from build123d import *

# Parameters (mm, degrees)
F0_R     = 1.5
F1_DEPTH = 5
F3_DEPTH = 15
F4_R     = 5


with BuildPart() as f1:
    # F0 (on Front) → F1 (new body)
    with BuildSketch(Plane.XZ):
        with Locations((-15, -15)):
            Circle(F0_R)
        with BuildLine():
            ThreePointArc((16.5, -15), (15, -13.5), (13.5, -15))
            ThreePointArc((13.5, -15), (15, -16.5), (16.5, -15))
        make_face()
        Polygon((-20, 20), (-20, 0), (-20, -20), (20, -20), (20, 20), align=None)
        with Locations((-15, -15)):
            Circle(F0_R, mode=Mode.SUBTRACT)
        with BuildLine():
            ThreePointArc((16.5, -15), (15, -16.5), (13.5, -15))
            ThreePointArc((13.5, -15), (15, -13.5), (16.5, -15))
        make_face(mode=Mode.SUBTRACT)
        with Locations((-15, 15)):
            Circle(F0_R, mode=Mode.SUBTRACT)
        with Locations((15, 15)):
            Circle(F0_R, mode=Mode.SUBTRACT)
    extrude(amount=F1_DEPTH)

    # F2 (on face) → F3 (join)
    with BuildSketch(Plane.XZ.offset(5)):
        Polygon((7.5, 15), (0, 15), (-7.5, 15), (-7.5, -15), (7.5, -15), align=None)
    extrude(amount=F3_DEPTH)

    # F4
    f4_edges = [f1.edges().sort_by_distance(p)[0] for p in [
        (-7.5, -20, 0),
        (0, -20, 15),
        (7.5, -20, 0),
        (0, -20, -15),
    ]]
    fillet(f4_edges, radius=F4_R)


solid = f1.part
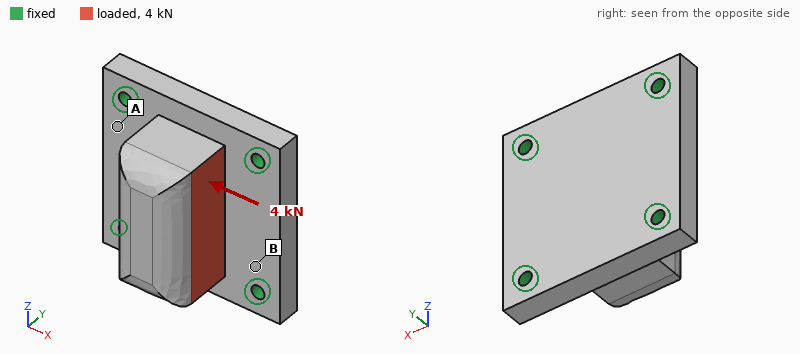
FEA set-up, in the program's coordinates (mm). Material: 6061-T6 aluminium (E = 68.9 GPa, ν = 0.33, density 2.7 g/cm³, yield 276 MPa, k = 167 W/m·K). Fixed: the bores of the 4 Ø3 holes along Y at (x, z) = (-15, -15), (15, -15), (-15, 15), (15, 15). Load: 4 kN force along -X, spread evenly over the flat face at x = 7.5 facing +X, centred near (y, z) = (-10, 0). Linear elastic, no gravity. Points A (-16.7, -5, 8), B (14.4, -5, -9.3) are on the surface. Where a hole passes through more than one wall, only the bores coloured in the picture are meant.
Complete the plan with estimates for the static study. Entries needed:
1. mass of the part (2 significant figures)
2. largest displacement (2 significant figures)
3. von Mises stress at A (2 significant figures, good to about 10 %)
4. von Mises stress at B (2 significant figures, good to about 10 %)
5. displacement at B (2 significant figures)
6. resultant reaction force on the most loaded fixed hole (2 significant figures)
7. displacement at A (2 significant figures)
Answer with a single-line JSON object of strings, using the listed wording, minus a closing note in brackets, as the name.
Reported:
{"mass of the part": "38 g", "largest displacement": "21 µm", "von Mises stress at A": "6.8 MPa", "von Mises stress at B": "13 MPa", "displacement at B": "3.9 µm", "resultant reaction force on the most loaded fixed hole": "1.2 kN", "displacement at A": "3.9 µm"}
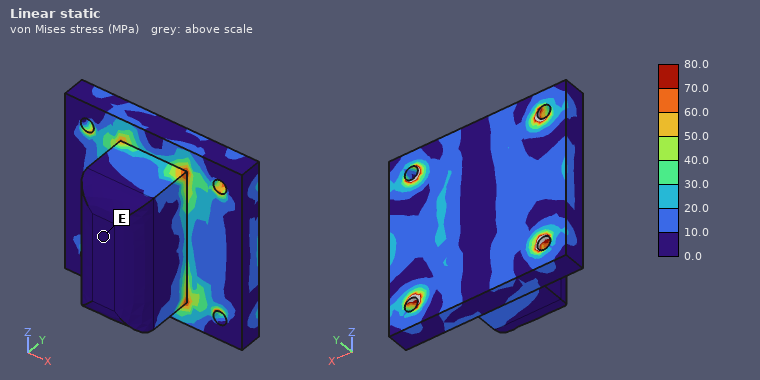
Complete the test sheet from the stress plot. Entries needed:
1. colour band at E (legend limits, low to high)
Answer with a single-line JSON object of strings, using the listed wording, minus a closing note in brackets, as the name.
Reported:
{"colour band at E": "0.0 to 10.0 MPa"}
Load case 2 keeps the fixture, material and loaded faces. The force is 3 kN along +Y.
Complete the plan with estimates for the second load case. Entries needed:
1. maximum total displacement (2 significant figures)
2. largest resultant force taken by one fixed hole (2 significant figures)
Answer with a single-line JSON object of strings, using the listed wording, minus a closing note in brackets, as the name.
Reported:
{"maximum total displacement": "24 µm", "largest resultant force taken by one fixed hole": "1.2 kN"}
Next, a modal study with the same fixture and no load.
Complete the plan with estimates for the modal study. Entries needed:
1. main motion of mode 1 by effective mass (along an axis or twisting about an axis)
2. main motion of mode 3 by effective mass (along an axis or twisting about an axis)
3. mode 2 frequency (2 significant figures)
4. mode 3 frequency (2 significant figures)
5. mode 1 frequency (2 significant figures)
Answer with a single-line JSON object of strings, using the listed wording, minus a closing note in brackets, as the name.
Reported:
{"main motion of mode 1 by effective mass": "along Y", "main motion of mode 3 by effective mass": "along X", "mode 2 frequency": "15 kHz", "mode 3 frequency": "16 kHz", "mode 1 frequency": "14 kHz"}
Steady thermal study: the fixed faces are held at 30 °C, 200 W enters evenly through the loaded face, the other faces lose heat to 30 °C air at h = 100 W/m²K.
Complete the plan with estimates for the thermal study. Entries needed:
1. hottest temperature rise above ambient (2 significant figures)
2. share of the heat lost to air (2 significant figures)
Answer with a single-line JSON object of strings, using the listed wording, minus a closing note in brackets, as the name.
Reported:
{"hottest temperature rise above ambient": "71 K", "share of the heat lost to air": "7.1 %"}
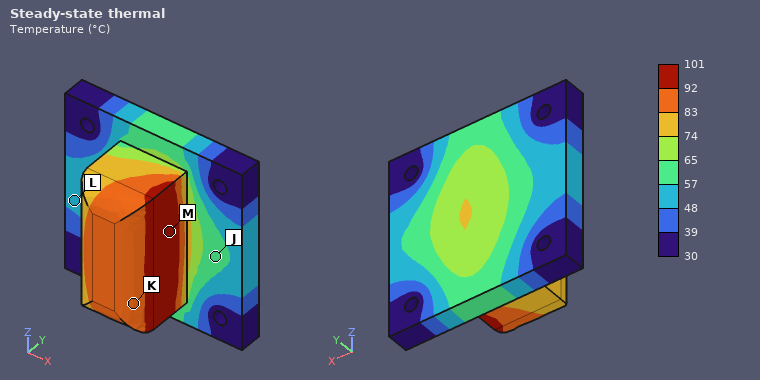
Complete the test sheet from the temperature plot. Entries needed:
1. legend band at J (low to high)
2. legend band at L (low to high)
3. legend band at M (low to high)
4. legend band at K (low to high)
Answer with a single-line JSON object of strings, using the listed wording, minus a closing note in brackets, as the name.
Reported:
{"legend band at J": "57 to 65 °C", "legend band at L": "48 to 57 °C", "legend band at M": "92 to 101 °C", "legend band at K": "83 to 92 °C"}
